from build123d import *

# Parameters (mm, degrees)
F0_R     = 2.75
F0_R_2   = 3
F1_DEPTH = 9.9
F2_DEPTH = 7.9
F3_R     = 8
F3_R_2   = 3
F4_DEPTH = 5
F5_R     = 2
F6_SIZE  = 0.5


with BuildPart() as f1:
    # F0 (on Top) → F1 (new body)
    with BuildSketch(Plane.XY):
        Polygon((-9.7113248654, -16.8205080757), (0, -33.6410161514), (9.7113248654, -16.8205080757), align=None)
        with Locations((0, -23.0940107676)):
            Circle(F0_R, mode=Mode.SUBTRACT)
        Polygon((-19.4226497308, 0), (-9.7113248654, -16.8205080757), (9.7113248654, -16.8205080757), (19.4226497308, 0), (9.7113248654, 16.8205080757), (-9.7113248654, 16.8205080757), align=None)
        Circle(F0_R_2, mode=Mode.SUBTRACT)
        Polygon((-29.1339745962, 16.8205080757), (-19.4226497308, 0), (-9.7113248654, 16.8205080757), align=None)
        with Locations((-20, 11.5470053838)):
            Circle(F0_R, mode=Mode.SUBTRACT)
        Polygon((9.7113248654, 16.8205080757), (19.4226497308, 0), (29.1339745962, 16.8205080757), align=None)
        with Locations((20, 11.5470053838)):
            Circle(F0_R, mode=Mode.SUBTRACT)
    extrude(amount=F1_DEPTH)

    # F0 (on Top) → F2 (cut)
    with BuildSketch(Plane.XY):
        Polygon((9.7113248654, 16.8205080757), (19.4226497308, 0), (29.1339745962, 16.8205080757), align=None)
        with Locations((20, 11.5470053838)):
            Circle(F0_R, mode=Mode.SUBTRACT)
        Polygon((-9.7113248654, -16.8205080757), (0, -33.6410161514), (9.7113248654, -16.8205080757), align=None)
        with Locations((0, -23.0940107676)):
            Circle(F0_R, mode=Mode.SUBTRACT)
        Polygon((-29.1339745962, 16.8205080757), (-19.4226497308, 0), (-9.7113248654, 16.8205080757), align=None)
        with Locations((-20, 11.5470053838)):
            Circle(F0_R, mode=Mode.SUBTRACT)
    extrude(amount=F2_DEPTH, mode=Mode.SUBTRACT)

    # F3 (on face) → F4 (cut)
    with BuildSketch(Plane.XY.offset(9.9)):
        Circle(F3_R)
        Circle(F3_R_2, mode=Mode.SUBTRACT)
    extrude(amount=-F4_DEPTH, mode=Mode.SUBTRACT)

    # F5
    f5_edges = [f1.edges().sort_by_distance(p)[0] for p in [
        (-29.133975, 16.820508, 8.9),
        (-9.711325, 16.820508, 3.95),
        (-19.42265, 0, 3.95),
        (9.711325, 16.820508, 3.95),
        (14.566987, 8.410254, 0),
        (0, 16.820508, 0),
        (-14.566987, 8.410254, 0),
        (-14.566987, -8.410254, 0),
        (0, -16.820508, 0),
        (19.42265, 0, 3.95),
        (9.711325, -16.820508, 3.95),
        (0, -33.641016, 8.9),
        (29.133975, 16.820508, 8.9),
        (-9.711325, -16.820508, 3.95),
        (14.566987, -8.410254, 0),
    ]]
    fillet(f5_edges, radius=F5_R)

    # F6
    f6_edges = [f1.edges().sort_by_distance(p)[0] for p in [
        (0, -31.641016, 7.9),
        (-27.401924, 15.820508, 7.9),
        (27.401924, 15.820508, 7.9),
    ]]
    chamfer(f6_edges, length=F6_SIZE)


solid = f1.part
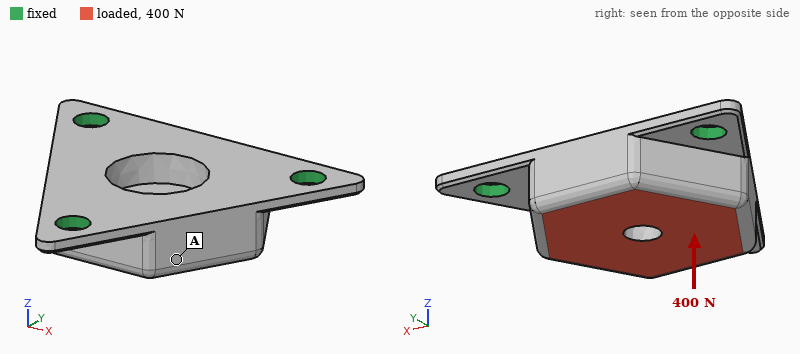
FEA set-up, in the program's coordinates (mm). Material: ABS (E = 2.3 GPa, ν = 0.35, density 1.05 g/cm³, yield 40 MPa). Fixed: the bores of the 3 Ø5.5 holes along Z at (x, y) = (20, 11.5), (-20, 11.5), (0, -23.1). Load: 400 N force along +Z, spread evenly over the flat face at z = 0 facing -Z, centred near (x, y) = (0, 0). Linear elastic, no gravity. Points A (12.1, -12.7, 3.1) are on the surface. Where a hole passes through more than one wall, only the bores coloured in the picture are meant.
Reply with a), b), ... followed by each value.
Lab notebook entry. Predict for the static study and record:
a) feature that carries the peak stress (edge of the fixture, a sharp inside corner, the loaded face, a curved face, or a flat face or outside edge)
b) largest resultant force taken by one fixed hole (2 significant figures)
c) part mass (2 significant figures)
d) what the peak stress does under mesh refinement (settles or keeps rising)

a) edge of the fixture
b) 170 N
c) 9.7 g
d) keeps rising
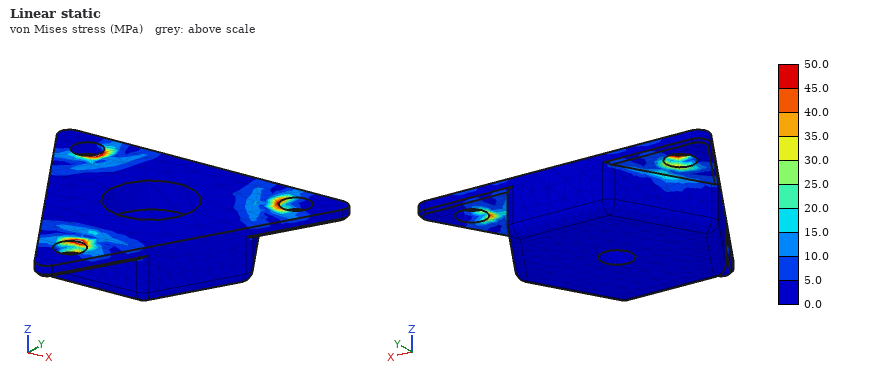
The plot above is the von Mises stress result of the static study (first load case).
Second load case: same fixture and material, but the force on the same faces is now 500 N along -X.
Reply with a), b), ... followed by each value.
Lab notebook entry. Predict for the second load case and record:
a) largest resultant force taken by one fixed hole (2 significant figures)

a) 260 N
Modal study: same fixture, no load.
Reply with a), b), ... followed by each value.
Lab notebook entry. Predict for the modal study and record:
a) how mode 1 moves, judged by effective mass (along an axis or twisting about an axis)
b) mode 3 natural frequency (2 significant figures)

a) along Z
b) 3600 Hz
